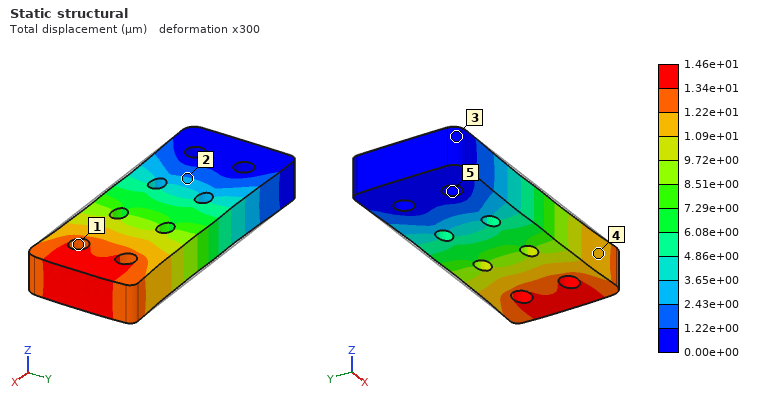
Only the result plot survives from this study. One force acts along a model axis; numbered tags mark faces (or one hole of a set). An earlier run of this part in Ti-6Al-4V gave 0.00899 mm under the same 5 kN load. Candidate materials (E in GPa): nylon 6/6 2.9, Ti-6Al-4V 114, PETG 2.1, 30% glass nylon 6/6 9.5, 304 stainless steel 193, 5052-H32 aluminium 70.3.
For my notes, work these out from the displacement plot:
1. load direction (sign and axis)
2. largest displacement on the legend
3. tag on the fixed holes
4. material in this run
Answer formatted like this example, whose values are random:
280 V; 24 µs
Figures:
+X; 1.46e+01 µm; 5; 5052-H32 aluminium
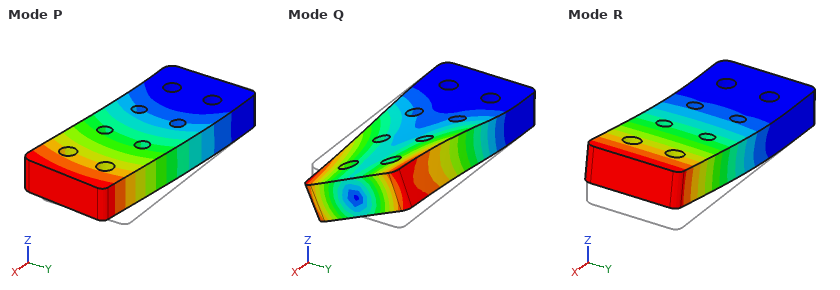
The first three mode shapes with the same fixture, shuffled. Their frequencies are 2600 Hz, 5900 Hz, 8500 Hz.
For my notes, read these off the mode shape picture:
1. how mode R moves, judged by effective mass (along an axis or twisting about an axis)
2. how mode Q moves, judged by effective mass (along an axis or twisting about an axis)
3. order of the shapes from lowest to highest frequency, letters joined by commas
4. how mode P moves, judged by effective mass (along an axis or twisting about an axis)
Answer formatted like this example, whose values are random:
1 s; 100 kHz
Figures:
along Z; twisting about X; R, P, Q; along Y
